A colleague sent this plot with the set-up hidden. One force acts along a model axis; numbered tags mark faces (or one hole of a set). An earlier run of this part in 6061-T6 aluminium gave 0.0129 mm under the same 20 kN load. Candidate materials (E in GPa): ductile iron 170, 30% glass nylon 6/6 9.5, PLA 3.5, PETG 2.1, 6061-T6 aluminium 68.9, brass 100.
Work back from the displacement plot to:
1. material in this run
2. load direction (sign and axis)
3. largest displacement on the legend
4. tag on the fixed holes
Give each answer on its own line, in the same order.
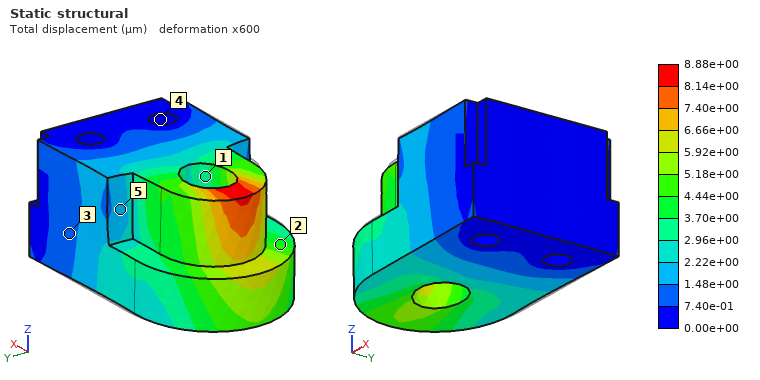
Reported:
brass
-X
8.88e+00 µm
4
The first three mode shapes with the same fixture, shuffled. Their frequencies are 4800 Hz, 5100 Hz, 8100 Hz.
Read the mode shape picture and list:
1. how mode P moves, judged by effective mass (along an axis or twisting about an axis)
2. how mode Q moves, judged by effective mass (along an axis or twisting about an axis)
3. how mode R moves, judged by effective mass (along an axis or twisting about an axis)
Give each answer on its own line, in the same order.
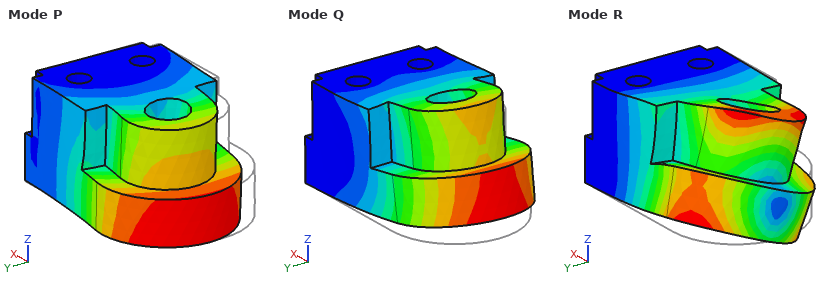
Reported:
along Y
along Z
twisting about X
